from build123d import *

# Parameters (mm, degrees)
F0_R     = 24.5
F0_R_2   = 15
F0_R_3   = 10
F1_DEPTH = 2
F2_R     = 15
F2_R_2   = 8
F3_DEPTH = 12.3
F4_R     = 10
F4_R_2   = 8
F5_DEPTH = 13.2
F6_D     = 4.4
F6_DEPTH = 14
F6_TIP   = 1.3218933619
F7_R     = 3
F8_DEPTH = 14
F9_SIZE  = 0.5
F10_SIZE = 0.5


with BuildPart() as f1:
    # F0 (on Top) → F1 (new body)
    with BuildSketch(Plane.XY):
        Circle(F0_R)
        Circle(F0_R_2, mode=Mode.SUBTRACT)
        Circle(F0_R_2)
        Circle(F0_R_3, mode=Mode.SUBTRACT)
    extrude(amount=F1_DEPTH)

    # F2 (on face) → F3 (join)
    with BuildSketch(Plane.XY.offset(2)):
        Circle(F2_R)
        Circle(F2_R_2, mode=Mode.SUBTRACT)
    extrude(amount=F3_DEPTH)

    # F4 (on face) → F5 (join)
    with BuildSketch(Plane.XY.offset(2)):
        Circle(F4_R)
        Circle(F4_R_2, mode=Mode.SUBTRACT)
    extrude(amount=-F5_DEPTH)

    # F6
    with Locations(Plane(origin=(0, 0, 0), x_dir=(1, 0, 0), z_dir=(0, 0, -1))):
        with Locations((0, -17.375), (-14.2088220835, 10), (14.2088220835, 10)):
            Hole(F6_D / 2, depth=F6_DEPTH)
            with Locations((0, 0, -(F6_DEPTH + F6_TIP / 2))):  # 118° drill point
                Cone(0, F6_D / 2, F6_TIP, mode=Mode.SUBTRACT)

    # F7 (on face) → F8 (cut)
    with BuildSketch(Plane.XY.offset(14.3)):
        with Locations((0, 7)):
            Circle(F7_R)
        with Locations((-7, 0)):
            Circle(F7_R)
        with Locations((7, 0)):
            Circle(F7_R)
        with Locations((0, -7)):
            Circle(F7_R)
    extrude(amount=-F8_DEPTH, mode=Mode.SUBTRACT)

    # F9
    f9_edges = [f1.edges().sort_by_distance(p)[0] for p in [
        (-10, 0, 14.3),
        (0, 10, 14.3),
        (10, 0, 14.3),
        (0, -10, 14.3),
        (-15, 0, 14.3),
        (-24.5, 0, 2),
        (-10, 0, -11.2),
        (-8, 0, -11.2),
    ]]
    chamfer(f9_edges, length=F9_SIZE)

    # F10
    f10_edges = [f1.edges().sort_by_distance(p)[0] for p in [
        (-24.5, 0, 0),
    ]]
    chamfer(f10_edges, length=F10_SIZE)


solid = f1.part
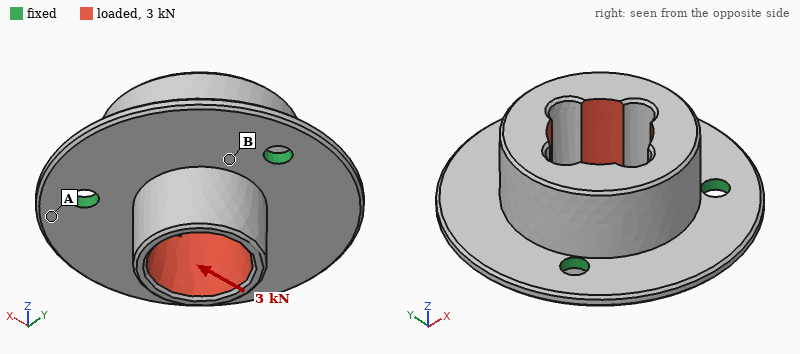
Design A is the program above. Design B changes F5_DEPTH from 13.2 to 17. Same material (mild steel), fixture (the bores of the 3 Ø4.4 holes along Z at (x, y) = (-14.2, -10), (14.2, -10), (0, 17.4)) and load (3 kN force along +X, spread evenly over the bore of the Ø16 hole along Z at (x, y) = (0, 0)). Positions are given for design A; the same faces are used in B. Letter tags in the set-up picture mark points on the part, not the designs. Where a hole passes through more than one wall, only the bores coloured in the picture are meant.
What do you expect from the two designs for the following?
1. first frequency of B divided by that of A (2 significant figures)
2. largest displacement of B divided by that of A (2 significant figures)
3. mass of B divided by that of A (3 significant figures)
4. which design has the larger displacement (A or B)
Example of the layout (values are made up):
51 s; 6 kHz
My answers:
0.98; 1.5; 1.04; B
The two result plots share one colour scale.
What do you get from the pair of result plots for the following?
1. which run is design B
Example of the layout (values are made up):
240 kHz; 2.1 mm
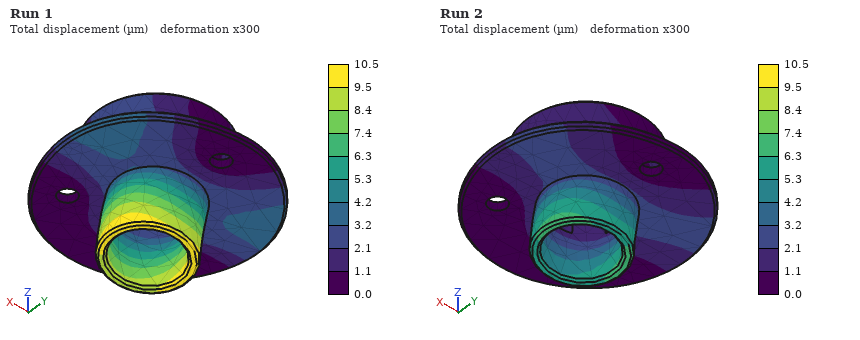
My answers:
Run 1
